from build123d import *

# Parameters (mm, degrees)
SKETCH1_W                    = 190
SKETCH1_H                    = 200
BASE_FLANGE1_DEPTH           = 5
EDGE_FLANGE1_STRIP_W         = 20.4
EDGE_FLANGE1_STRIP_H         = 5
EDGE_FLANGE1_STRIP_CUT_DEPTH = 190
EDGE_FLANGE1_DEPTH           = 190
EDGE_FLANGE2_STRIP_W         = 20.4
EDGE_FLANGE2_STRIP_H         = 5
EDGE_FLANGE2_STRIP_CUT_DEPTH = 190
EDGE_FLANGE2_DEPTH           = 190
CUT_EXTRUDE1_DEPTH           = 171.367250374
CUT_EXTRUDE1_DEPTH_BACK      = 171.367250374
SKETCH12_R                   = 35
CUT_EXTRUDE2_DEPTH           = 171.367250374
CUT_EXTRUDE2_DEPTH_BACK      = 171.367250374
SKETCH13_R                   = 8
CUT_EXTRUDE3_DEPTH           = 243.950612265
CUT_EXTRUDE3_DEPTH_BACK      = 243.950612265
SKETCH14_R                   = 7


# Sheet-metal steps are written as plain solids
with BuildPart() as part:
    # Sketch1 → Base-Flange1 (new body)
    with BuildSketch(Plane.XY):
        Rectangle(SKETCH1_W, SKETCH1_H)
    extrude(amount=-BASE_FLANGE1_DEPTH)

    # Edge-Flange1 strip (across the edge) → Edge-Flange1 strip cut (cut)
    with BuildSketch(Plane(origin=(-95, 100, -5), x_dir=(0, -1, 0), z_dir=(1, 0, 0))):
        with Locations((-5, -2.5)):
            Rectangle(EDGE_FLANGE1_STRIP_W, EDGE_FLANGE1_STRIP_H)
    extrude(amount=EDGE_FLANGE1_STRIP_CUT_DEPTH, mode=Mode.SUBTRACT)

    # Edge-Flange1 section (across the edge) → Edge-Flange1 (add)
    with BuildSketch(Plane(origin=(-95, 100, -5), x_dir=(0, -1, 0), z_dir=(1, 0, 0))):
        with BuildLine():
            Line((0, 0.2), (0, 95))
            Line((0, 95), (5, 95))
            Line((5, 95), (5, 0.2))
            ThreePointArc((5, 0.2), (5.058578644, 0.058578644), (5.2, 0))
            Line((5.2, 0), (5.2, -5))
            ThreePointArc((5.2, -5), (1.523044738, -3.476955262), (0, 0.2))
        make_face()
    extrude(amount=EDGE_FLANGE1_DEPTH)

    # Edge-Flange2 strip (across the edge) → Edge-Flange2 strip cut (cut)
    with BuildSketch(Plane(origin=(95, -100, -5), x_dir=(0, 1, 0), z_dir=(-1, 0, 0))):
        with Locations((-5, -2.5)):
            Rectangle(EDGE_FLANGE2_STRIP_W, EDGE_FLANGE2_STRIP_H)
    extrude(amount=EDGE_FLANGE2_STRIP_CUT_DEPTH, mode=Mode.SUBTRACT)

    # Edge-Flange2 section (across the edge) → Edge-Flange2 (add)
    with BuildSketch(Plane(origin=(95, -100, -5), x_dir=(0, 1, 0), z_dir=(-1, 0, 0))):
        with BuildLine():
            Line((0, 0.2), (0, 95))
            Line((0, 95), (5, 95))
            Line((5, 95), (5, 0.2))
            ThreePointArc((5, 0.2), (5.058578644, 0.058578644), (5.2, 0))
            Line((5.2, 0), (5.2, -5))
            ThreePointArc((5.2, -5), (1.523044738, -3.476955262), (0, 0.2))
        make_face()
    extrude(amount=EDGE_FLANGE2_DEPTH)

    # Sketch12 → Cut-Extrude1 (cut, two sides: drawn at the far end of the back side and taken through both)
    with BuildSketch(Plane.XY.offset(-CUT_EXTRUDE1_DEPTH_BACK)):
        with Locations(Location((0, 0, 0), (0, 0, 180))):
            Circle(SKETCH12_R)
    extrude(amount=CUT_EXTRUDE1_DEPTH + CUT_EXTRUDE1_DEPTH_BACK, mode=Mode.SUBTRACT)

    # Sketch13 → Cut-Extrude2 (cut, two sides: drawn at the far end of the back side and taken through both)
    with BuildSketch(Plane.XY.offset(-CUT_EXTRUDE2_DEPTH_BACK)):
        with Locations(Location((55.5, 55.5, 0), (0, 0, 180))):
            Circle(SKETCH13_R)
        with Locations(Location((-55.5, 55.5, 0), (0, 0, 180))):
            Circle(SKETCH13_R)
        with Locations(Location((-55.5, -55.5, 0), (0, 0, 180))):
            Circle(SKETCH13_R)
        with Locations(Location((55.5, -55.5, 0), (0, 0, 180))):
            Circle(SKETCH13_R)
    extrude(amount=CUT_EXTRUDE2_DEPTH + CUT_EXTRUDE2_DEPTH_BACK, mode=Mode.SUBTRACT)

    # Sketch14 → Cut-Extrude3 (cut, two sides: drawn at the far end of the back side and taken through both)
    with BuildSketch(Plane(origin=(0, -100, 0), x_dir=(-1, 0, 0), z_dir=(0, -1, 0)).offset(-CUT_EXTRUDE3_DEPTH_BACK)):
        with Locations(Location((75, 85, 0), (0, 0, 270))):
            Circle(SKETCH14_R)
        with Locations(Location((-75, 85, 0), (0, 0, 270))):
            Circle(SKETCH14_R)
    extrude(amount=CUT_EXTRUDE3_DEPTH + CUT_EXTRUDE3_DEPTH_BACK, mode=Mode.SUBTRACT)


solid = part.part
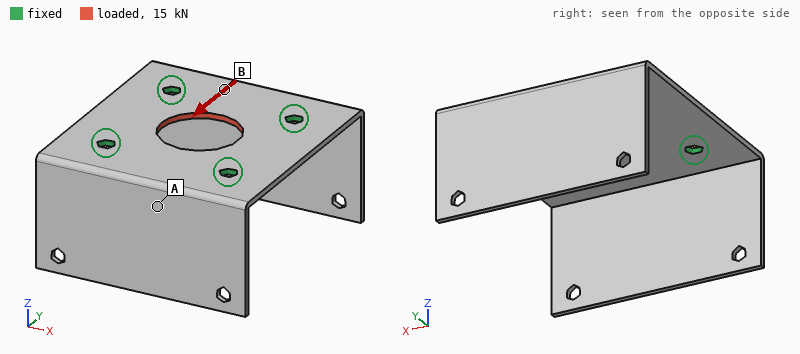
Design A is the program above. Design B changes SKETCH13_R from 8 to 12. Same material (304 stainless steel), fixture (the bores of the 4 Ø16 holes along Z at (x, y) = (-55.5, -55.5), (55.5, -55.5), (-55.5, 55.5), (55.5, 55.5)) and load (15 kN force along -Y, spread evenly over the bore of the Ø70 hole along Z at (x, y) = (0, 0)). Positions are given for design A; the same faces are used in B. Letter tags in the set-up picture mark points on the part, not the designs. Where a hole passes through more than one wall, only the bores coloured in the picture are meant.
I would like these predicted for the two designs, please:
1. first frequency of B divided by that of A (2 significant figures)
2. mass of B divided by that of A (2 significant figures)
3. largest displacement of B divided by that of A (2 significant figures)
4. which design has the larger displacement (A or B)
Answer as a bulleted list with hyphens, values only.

- 1.1
- 0.99
- 0.88
- A
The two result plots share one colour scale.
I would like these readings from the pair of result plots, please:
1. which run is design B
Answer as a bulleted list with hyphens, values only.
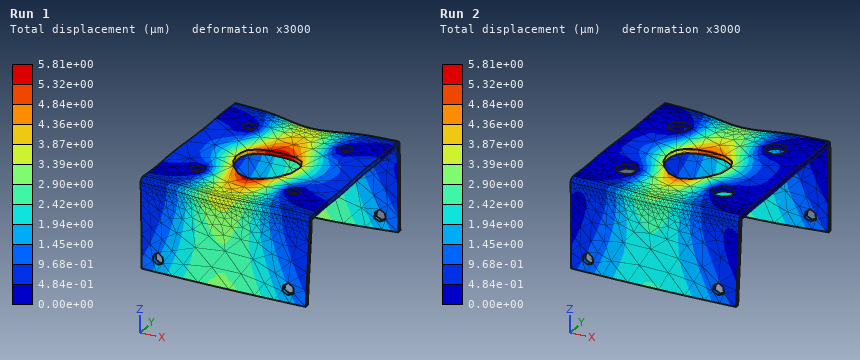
- Run 2
